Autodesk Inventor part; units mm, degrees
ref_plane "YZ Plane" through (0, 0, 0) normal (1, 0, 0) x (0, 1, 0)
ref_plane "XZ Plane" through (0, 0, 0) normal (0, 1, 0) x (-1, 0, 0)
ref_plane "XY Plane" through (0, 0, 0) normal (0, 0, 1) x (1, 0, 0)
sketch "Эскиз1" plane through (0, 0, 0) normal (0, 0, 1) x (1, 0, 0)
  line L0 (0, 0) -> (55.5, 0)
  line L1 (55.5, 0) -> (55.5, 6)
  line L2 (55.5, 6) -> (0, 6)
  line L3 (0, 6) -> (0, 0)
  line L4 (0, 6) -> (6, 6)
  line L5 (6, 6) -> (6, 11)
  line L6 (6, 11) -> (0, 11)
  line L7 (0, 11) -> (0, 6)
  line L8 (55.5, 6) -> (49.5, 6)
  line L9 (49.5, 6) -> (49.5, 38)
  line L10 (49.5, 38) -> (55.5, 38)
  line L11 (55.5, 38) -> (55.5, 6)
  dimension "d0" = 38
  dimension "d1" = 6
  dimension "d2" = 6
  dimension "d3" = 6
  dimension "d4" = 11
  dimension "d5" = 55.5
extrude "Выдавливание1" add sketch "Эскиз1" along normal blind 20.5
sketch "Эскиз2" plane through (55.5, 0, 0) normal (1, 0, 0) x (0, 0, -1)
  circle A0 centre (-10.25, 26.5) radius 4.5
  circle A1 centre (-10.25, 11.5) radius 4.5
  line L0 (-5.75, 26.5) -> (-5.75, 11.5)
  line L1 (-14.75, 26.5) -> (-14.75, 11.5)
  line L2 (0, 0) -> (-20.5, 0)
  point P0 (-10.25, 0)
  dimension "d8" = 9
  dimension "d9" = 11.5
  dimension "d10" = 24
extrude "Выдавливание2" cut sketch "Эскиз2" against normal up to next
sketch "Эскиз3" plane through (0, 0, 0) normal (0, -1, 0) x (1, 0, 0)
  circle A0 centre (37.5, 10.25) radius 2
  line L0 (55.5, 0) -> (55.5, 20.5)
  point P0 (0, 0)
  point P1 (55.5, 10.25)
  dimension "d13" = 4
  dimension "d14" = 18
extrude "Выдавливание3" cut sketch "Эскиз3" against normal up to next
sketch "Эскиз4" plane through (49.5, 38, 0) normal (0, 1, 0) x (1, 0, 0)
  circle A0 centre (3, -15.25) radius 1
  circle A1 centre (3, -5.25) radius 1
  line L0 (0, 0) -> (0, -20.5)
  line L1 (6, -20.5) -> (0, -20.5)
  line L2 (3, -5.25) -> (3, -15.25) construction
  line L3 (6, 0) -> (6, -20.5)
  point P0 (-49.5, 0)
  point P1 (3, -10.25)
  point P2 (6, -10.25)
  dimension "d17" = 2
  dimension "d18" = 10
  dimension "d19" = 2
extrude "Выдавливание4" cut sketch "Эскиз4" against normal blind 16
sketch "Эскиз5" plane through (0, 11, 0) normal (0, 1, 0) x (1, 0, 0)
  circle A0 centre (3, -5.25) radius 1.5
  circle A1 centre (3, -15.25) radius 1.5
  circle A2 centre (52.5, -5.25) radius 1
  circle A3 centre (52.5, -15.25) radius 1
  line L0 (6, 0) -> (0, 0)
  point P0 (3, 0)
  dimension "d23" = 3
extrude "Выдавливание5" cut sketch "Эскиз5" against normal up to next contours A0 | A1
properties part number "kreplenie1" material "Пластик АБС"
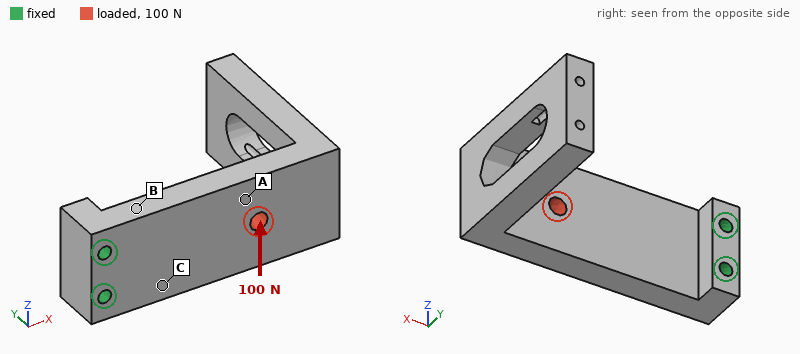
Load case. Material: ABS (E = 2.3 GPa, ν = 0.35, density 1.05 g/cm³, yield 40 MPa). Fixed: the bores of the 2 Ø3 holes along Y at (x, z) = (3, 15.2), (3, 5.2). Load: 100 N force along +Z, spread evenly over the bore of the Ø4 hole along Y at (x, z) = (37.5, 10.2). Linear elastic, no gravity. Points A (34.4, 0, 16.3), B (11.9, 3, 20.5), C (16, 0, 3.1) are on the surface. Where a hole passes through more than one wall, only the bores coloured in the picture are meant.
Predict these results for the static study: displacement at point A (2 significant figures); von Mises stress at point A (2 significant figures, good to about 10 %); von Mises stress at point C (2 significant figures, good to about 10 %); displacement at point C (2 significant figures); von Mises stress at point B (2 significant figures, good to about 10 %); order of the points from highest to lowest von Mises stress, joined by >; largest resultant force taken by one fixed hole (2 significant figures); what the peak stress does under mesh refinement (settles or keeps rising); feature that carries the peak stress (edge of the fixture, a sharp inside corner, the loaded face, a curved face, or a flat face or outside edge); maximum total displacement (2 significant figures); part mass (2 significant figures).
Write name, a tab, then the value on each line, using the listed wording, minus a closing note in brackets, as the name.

displacement at point A	0.18 mm
von Mises stress at point A	1.5 MPa
von Mises stress at point C	3.6 MPa
displacement at point C	0.057 mm
von Mises stress at point B	5.7 MPa
order of the points from highest to lowest von Mises stress, joined by >	B > C > A
largest resultant force taken by one fixed hole	270 N
what the peak stress does under mesh refinement	keeps rising
feature that carries the peak stress	edge of the fixture
maximum total displacement	0.35 mm
part mass	10 g
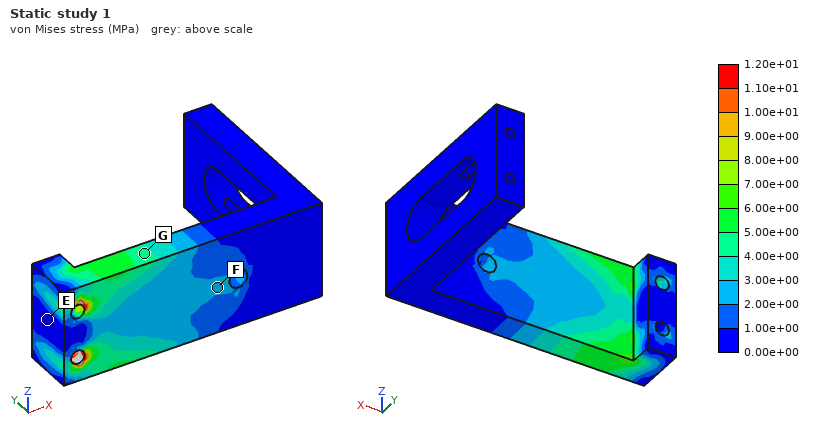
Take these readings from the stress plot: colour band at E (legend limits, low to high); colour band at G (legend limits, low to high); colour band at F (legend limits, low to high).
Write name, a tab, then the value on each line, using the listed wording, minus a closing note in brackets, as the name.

colour band at E	0.00e+00 to 1.00e+00 MPa
colour band at G	4.00e+00 to 5.00e+00 MPa
colour band at F	2.00e+00 to 3.00e+00 MPa
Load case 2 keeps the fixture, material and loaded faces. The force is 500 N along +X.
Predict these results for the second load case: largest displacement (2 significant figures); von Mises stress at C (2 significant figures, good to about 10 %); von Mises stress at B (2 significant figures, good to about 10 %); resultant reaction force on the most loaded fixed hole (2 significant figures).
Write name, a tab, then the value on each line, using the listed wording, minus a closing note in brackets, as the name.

largest displacement	82 µm
von Mises stress at C	4.0 MPa
von Mises stress at B	3.5 MPa
resultant reaction force on the most loaded fixed hole	250 N
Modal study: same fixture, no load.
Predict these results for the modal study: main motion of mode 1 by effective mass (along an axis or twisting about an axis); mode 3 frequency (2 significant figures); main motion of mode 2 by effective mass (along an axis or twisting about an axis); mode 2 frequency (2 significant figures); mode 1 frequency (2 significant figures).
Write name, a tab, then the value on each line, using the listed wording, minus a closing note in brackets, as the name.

main motion of mode 1 by effective mass	along Y
mode 3 frequency	860 Hz
main motion of mode 2 by effective mass	along Z
mode 2 frequency	540 Hz
mode 1 frequency	300 Hz
